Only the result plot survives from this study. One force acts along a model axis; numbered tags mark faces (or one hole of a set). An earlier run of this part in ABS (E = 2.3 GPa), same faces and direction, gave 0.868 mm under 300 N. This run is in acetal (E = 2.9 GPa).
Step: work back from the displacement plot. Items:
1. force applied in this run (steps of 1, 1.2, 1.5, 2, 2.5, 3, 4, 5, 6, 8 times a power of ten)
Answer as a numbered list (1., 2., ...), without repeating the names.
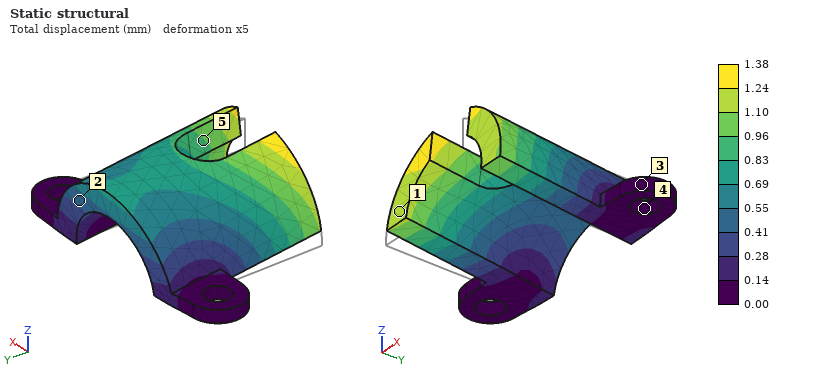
1. 600 N
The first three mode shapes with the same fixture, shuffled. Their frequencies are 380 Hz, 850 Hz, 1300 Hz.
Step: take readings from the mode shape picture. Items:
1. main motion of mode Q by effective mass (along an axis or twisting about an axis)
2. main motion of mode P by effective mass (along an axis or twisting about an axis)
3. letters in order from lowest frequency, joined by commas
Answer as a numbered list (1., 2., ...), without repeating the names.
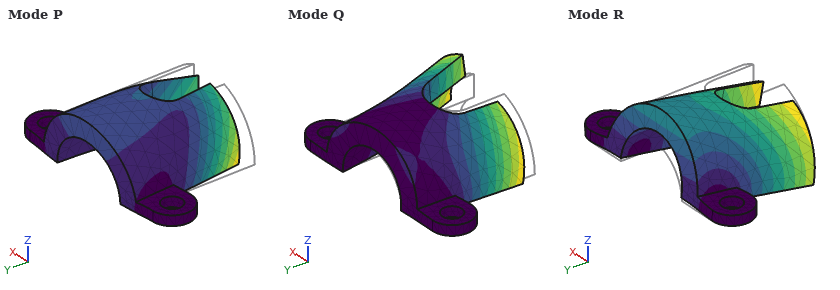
1. along X
2. along Y
3. R, Q, P
